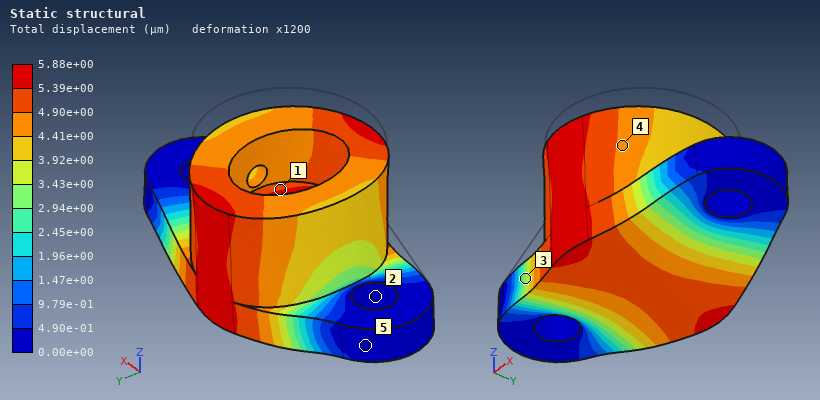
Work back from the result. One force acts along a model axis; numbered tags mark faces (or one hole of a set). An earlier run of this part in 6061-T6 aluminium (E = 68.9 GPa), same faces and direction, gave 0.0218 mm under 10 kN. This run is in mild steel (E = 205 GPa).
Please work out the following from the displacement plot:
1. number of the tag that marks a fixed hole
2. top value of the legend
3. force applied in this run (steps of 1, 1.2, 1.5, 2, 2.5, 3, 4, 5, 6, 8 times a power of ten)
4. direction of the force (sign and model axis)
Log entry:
2
5.88e+00 µm
8 kN
-Z
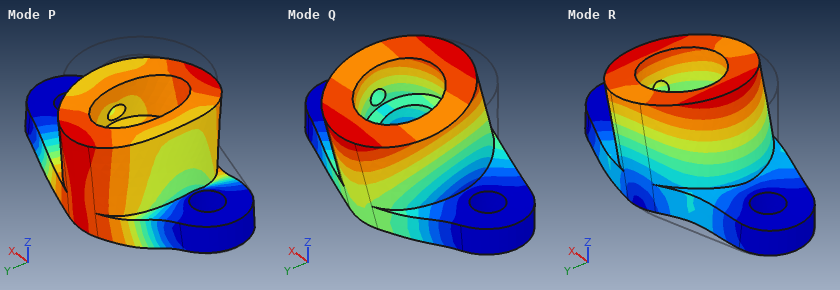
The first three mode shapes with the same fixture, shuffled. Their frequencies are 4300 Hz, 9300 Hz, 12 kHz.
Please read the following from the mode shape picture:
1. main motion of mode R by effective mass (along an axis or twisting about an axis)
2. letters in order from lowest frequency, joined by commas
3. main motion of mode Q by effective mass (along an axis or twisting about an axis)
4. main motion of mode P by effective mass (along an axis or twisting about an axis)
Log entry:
along X
Q, P, R
along Y
along Z
